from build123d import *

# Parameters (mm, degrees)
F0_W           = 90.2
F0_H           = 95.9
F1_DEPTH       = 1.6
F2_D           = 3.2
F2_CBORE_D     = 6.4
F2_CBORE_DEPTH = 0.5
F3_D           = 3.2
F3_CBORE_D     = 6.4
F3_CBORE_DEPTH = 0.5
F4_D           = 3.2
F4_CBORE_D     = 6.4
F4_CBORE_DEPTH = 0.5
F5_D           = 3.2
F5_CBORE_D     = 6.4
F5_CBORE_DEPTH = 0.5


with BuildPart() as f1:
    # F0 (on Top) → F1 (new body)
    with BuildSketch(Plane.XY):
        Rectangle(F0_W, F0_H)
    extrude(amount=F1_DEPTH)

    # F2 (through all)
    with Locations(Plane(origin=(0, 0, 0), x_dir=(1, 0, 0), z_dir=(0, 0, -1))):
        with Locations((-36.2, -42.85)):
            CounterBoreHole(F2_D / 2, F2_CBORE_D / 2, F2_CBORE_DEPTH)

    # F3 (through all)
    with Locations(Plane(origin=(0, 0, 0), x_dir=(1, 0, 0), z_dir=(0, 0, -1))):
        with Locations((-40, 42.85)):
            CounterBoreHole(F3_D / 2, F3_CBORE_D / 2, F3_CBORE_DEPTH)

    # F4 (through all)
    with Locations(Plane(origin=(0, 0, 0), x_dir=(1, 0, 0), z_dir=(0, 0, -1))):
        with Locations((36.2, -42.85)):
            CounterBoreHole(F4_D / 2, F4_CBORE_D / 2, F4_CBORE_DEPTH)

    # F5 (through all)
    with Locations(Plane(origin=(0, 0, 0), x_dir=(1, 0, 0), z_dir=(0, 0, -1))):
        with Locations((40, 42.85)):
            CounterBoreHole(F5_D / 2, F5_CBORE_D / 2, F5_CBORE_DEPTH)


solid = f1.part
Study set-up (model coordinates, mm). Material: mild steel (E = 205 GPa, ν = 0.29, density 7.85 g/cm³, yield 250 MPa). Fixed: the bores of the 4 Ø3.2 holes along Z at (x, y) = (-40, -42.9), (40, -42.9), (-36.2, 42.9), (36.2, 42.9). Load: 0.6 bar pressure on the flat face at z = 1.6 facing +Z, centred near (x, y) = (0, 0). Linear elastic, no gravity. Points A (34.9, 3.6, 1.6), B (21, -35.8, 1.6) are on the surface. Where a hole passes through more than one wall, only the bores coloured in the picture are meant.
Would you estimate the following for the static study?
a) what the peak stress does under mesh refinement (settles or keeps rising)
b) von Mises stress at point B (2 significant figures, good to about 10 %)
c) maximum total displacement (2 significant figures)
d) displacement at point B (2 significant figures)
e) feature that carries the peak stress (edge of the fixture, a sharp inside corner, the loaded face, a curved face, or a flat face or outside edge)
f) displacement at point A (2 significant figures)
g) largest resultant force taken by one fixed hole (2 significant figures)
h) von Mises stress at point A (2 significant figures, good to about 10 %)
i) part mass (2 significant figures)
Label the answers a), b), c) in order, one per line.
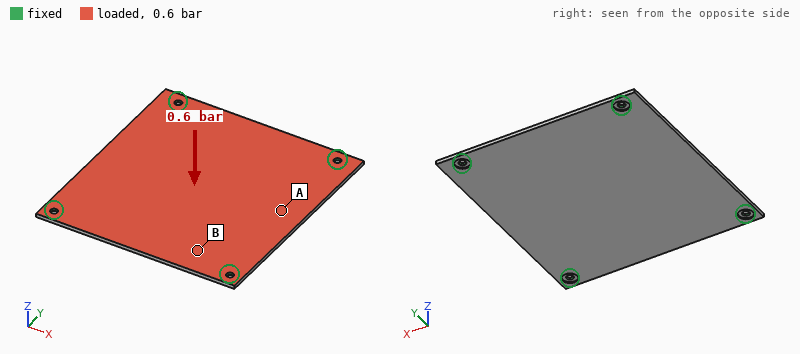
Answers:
a) keeps rising
b) 25 MPa
c) 0.32 mm
d) 0.14 mm
e) edge of the fixture
f) 0.23 mm
g) 260 N
h) 58 MPa
i) 110 g
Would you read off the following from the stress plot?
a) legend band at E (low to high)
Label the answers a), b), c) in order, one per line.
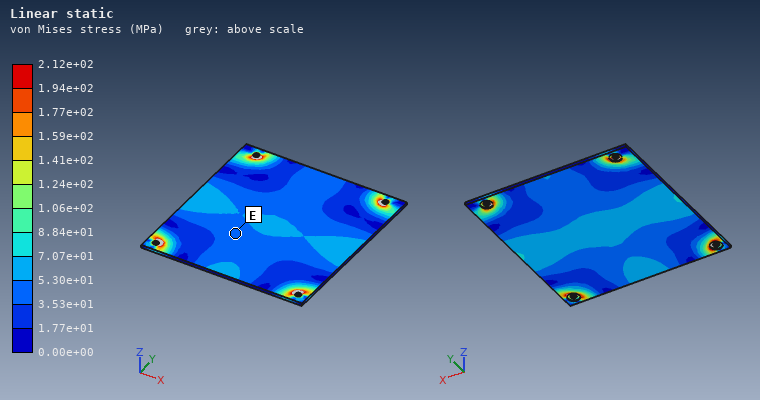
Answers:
a) 3.53e+01 to 5.30e+01 MPa
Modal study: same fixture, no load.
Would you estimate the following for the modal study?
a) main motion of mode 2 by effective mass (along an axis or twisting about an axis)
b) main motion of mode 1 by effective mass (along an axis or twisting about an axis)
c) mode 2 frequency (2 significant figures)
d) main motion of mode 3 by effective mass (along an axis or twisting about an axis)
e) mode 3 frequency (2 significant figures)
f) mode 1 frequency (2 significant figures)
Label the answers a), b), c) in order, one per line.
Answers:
a) twisting about Y
b) along Z
c) 1200 Hz
d) twisting about X
e) 1400 Hz
f) 740 Hz
